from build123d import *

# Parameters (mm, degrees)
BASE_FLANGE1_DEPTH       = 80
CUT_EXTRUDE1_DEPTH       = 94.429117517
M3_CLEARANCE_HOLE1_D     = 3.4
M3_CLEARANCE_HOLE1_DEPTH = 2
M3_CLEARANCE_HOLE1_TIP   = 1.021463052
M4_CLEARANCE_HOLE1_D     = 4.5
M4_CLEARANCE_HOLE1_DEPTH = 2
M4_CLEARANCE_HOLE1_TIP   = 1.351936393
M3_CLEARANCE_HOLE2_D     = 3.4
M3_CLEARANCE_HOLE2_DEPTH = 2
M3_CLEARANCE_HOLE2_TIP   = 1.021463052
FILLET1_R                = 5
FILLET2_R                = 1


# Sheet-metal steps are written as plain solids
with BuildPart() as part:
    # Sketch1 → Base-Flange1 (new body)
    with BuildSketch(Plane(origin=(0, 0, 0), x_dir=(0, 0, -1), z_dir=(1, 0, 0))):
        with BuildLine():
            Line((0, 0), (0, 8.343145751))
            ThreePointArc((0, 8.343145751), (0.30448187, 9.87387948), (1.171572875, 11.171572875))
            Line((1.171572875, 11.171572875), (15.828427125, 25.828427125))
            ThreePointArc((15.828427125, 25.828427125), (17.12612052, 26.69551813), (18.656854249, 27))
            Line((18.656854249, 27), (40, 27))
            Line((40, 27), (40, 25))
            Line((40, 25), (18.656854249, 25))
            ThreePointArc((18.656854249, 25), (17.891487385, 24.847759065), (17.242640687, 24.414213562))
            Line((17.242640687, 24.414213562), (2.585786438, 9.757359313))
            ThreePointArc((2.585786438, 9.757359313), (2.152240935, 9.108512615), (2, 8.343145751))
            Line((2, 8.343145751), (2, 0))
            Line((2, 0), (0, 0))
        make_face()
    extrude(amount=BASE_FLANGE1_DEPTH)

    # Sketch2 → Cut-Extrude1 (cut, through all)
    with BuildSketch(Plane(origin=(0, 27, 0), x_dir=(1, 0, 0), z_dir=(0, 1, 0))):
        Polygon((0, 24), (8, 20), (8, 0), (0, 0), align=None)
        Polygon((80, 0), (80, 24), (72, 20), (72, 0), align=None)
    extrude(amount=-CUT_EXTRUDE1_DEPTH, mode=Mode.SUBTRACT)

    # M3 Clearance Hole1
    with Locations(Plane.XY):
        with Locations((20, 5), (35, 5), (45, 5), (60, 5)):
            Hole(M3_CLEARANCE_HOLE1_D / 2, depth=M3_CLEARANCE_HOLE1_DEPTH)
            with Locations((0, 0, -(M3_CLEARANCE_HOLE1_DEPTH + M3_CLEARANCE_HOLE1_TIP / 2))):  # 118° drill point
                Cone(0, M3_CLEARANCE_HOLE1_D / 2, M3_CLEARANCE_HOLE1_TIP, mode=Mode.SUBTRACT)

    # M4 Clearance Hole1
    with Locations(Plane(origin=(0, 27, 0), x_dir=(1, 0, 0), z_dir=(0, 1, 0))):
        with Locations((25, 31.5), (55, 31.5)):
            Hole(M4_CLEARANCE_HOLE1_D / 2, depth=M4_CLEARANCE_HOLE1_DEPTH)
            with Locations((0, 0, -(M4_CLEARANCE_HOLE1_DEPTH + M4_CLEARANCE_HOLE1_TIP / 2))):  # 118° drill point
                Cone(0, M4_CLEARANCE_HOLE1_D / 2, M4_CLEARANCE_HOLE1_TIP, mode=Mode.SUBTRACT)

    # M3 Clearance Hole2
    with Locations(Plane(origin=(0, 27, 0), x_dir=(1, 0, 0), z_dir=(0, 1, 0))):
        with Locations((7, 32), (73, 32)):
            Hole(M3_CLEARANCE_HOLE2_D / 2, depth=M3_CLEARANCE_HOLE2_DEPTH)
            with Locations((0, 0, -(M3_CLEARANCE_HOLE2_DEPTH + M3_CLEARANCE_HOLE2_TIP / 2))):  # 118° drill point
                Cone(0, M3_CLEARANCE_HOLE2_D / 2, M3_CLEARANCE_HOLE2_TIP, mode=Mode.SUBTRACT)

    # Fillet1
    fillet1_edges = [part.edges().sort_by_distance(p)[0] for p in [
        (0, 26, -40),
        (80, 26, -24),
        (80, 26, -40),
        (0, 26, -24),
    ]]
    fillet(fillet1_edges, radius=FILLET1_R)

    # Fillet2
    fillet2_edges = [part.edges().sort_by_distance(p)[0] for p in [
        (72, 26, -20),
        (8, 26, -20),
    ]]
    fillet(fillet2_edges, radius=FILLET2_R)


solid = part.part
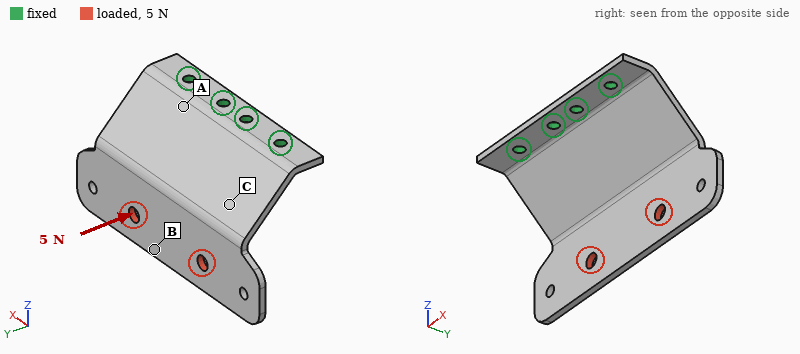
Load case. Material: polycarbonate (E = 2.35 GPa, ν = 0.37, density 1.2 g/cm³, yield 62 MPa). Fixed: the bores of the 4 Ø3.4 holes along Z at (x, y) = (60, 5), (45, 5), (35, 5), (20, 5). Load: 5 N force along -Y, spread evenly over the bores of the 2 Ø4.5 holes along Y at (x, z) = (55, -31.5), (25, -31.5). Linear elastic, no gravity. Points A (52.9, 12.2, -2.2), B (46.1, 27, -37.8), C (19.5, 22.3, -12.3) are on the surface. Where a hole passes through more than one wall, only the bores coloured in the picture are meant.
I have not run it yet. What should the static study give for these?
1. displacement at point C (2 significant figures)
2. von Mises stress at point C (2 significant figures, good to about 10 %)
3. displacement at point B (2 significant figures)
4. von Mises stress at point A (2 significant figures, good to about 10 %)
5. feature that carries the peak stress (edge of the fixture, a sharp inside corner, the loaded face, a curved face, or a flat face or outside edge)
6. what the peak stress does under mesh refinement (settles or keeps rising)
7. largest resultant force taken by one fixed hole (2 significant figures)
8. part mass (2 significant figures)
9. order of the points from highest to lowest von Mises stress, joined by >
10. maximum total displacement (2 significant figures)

0.28 mm
1.8 MPa
1.0 mm
2.9 MPa
edge of the fixture
keeps rising
2.1 N
8.9 g
A > C > B
1.1 mm
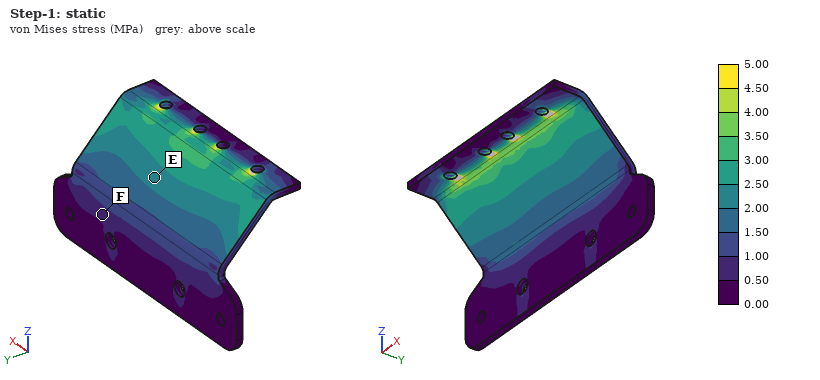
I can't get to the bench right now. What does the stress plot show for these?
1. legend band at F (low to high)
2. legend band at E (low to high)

0.50 to 1.00 MPa
2.00 to 2.50 MPa
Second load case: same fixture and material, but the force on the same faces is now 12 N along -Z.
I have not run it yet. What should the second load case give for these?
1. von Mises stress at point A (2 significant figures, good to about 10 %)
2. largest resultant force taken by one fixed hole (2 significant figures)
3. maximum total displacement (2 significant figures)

3.5 MPa
3.4 N
1.1 mm
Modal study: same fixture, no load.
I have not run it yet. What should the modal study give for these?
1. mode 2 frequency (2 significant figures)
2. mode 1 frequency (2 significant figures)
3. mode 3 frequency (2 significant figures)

300 Hz
190 Hz
870 Hz
